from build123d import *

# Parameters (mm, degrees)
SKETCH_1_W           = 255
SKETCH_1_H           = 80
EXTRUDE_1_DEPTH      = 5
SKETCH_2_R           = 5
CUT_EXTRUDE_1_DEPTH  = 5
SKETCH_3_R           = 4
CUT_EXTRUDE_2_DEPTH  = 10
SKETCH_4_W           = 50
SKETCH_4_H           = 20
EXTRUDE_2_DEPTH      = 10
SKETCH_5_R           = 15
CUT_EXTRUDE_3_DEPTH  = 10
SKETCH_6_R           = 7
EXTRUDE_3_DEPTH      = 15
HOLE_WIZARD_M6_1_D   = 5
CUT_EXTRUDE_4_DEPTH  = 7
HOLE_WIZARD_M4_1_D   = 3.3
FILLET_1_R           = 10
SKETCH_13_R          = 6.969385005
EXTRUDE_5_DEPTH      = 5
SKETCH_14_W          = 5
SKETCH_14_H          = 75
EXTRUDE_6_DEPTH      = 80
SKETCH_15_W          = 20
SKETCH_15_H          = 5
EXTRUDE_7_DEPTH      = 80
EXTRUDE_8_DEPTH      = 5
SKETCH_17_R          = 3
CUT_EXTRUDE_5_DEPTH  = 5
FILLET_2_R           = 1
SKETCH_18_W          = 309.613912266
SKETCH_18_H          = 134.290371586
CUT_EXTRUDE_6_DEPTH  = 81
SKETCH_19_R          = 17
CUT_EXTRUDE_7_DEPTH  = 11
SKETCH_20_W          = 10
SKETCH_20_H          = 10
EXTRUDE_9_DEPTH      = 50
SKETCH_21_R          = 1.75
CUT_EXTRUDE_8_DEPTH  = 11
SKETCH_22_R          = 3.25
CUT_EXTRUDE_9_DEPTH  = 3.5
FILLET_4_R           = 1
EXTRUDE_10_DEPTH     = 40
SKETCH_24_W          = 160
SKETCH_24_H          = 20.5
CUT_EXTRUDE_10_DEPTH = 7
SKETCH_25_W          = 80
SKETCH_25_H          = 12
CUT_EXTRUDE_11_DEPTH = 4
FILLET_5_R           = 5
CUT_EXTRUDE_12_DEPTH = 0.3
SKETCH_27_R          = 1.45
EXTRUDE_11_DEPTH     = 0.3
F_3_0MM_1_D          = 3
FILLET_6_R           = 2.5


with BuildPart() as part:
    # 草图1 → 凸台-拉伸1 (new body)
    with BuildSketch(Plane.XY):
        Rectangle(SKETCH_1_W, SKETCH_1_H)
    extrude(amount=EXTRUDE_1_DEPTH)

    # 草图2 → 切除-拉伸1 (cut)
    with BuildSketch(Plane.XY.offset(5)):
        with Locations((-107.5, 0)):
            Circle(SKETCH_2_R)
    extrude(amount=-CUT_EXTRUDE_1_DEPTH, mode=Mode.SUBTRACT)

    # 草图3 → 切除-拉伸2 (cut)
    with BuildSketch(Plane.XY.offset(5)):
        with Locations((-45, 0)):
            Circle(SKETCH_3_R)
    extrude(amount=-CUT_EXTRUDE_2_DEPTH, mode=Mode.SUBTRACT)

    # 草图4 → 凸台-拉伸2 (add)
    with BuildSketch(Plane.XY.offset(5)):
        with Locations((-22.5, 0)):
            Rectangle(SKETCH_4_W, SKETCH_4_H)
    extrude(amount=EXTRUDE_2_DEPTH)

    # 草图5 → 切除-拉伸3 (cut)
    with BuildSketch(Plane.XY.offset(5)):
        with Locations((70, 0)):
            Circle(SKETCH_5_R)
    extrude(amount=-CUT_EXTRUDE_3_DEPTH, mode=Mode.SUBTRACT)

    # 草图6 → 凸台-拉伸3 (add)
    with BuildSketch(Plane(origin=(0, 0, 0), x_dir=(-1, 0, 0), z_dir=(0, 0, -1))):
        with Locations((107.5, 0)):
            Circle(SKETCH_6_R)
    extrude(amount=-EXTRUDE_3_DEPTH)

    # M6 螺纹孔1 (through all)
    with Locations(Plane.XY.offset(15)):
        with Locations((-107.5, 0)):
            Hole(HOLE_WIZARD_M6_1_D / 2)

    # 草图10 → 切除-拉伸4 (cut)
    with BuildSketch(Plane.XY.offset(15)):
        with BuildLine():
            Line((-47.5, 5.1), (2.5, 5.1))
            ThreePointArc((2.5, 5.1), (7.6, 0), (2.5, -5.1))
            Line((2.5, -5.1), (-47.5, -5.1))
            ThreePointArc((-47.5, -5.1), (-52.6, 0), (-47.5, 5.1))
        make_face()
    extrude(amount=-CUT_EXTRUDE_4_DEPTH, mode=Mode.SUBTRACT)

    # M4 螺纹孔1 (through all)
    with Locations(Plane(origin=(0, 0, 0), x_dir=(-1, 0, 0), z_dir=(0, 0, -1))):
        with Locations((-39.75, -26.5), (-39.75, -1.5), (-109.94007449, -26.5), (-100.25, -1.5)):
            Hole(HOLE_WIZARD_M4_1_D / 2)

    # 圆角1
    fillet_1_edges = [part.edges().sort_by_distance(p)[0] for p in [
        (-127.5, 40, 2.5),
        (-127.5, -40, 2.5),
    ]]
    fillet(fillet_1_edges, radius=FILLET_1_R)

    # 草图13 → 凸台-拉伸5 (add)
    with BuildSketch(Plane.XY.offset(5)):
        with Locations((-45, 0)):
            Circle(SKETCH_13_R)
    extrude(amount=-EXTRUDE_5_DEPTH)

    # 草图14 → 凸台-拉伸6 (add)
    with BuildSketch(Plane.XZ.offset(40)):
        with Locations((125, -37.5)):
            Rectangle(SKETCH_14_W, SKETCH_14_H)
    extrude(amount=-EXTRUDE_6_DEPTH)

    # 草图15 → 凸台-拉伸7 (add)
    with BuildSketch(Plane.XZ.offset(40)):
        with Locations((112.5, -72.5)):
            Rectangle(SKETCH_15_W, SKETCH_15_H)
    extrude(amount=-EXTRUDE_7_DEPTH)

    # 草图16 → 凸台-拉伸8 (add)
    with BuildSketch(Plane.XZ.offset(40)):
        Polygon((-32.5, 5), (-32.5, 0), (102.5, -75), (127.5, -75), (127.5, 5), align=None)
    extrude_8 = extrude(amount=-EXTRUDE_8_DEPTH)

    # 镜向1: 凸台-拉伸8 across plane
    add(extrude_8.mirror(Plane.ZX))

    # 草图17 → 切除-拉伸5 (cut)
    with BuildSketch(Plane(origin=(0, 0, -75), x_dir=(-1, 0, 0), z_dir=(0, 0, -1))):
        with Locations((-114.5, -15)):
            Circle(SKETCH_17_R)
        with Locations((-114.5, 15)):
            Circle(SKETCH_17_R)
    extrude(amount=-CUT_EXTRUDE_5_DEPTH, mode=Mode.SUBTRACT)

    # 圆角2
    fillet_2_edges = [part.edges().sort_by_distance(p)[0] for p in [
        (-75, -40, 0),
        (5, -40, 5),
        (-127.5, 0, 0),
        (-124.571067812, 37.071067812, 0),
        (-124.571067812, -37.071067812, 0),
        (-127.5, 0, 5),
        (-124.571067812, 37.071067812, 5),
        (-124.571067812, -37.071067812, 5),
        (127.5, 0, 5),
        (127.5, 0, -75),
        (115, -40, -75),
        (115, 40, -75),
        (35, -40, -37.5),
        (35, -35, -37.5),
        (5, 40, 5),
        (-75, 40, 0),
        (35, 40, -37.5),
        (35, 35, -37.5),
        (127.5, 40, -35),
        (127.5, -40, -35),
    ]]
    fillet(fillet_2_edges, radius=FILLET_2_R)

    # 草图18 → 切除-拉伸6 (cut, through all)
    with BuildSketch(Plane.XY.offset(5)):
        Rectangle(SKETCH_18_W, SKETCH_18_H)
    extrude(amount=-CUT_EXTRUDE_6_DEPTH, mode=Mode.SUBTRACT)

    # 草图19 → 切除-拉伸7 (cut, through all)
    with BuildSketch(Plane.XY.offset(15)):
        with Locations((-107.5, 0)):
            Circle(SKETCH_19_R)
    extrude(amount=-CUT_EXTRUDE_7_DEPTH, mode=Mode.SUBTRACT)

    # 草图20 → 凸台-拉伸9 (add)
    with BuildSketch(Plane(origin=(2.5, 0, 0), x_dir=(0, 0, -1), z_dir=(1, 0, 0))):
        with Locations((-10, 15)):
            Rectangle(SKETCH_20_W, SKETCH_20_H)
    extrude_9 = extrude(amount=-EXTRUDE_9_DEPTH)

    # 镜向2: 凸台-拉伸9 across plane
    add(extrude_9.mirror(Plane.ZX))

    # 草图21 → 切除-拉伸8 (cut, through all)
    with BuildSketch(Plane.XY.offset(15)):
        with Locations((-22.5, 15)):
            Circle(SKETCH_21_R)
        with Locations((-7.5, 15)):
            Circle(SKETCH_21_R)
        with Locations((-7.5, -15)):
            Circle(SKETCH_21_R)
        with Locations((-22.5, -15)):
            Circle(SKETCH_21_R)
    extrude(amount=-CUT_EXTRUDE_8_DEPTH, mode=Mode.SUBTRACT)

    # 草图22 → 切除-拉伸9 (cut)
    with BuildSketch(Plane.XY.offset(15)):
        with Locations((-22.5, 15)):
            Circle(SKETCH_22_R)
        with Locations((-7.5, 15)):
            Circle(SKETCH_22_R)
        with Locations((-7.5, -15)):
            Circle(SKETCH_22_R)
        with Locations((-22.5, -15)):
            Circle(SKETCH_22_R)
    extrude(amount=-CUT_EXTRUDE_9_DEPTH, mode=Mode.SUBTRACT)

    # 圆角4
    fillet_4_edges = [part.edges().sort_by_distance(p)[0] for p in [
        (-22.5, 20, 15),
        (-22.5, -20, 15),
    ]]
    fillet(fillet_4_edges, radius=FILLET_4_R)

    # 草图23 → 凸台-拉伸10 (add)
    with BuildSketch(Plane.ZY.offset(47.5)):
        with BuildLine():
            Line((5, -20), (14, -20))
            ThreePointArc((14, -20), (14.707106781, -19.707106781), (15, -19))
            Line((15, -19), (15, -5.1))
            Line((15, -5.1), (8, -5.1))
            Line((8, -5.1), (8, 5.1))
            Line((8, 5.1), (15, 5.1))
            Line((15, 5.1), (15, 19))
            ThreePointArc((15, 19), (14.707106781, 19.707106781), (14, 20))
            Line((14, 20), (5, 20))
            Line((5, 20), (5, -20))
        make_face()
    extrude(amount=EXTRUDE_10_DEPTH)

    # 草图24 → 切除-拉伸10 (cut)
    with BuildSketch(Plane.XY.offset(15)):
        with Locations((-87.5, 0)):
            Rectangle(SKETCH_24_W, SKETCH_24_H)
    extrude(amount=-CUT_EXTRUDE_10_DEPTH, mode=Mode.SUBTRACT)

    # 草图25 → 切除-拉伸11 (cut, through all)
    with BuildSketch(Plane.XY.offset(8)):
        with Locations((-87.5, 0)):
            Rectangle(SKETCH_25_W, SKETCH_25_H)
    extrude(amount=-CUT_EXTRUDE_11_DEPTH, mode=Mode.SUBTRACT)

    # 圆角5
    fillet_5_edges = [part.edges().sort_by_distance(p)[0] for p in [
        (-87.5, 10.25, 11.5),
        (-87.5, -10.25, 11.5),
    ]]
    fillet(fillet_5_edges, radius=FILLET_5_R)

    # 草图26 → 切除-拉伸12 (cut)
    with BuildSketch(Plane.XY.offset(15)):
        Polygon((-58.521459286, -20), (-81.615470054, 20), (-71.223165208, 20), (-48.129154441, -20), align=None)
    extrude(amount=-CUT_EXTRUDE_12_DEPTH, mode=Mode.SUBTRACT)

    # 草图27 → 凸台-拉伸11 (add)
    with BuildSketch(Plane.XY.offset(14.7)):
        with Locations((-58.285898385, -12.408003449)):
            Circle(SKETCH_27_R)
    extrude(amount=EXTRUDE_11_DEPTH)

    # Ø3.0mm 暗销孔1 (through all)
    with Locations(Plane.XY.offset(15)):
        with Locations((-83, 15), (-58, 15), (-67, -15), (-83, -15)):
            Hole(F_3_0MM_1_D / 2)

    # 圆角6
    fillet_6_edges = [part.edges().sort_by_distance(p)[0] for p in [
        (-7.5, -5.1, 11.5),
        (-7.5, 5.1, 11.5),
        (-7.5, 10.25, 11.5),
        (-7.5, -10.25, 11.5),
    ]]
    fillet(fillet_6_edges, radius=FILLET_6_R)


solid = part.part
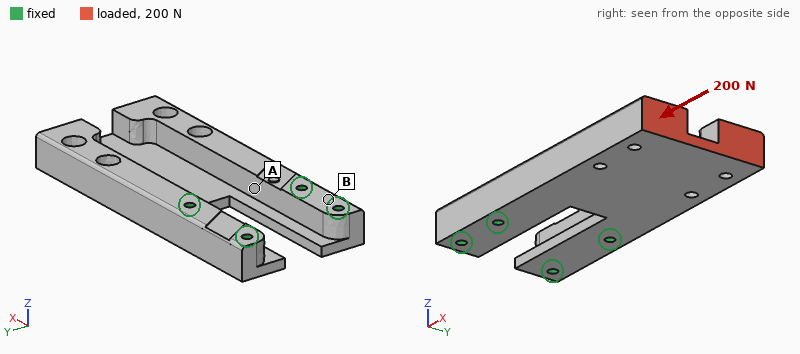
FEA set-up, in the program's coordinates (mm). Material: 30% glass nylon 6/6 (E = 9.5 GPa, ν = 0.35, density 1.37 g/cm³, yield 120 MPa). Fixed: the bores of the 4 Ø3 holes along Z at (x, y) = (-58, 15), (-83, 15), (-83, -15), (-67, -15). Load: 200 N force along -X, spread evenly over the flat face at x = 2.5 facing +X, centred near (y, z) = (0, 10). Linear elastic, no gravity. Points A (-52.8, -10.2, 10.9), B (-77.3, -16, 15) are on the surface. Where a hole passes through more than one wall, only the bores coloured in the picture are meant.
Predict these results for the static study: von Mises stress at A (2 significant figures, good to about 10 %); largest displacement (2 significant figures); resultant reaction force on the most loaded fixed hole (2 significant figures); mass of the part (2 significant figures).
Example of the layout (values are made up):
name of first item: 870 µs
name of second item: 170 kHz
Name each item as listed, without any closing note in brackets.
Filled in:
von Mises stress at A: 0.93 MPa
largest displacement: 15 µm
resultant reaction force on the most loaded fixed hole: 93 N
mass of the part: 29 g
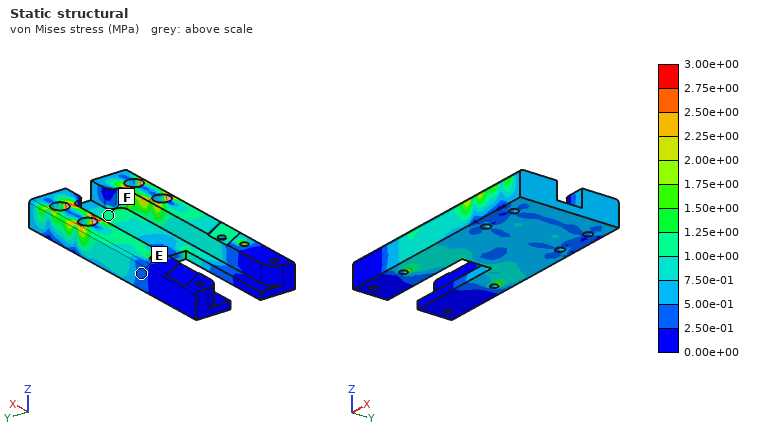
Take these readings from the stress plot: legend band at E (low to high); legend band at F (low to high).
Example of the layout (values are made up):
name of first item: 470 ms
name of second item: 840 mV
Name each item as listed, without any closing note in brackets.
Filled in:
legend band at E: 2.50e-01 to 5.00e-01 MPa
legend band at F: 1.00e+00 to 1.25e+00 MPa
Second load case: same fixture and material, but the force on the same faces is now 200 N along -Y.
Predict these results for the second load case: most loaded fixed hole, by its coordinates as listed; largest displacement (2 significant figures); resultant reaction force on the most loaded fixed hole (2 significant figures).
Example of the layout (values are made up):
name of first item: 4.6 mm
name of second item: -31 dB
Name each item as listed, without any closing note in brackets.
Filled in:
most loaded fixed hole, by its coordinates as listed: (-58, 15)
largest displacement: 0.18 mm
resultant reaction force on the most loaded fixed hole: 380 N
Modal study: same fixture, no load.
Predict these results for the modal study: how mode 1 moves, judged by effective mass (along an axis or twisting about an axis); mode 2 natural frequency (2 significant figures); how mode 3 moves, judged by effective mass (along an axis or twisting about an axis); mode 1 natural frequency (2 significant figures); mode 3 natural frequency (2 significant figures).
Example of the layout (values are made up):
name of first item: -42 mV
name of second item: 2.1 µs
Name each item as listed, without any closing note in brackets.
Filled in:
how mode 1 moves, judged by effective mass: along Z
mode 2 natural frequency: 1800 Hz
how mode 3 moves, judged by effective mass: along Y
mode 1 natural frequency: 890 Hz
mode 3 natural frequency: 2900 Hz
